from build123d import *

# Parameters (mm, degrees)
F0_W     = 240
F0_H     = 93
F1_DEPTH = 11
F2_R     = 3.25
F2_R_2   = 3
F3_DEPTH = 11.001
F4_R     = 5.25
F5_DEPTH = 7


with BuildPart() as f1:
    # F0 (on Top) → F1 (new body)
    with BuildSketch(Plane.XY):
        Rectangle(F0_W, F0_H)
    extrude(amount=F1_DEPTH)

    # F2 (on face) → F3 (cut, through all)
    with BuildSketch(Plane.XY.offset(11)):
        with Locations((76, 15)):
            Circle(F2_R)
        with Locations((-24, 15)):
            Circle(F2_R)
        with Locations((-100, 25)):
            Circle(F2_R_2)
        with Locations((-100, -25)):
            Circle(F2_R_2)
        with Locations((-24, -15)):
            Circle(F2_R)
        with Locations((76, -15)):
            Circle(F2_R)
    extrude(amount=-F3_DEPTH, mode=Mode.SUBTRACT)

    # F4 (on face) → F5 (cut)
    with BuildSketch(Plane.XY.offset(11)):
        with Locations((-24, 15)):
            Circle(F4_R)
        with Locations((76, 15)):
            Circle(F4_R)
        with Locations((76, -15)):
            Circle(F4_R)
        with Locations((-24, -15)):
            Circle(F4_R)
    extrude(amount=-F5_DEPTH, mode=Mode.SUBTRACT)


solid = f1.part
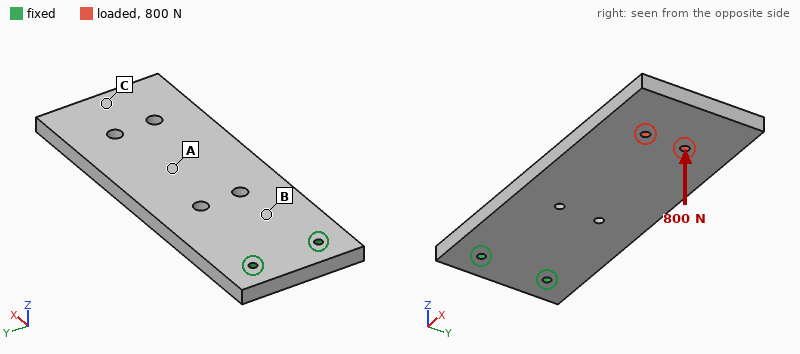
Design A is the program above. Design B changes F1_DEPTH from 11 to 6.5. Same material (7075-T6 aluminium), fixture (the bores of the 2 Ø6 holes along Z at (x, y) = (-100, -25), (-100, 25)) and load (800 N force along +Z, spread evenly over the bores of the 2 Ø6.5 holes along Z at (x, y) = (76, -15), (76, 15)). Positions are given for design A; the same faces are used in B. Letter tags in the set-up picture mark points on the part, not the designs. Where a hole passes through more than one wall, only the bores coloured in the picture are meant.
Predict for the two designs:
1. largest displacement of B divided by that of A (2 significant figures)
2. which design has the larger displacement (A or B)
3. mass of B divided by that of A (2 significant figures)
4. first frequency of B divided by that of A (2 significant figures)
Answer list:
4.7
B
0.59
0.60
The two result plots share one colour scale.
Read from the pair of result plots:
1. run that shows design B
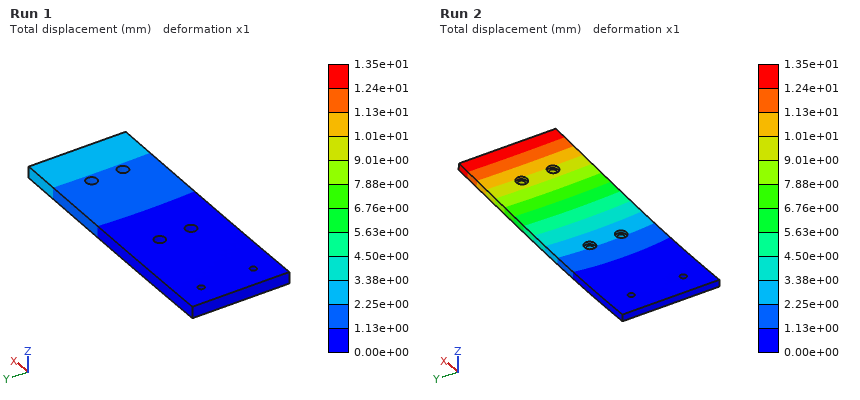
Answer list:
Run 2
